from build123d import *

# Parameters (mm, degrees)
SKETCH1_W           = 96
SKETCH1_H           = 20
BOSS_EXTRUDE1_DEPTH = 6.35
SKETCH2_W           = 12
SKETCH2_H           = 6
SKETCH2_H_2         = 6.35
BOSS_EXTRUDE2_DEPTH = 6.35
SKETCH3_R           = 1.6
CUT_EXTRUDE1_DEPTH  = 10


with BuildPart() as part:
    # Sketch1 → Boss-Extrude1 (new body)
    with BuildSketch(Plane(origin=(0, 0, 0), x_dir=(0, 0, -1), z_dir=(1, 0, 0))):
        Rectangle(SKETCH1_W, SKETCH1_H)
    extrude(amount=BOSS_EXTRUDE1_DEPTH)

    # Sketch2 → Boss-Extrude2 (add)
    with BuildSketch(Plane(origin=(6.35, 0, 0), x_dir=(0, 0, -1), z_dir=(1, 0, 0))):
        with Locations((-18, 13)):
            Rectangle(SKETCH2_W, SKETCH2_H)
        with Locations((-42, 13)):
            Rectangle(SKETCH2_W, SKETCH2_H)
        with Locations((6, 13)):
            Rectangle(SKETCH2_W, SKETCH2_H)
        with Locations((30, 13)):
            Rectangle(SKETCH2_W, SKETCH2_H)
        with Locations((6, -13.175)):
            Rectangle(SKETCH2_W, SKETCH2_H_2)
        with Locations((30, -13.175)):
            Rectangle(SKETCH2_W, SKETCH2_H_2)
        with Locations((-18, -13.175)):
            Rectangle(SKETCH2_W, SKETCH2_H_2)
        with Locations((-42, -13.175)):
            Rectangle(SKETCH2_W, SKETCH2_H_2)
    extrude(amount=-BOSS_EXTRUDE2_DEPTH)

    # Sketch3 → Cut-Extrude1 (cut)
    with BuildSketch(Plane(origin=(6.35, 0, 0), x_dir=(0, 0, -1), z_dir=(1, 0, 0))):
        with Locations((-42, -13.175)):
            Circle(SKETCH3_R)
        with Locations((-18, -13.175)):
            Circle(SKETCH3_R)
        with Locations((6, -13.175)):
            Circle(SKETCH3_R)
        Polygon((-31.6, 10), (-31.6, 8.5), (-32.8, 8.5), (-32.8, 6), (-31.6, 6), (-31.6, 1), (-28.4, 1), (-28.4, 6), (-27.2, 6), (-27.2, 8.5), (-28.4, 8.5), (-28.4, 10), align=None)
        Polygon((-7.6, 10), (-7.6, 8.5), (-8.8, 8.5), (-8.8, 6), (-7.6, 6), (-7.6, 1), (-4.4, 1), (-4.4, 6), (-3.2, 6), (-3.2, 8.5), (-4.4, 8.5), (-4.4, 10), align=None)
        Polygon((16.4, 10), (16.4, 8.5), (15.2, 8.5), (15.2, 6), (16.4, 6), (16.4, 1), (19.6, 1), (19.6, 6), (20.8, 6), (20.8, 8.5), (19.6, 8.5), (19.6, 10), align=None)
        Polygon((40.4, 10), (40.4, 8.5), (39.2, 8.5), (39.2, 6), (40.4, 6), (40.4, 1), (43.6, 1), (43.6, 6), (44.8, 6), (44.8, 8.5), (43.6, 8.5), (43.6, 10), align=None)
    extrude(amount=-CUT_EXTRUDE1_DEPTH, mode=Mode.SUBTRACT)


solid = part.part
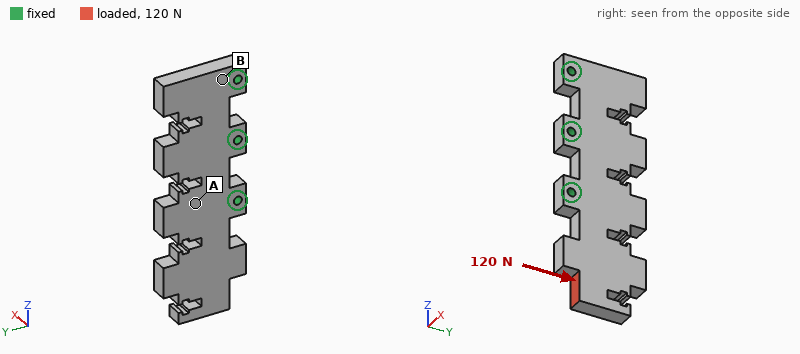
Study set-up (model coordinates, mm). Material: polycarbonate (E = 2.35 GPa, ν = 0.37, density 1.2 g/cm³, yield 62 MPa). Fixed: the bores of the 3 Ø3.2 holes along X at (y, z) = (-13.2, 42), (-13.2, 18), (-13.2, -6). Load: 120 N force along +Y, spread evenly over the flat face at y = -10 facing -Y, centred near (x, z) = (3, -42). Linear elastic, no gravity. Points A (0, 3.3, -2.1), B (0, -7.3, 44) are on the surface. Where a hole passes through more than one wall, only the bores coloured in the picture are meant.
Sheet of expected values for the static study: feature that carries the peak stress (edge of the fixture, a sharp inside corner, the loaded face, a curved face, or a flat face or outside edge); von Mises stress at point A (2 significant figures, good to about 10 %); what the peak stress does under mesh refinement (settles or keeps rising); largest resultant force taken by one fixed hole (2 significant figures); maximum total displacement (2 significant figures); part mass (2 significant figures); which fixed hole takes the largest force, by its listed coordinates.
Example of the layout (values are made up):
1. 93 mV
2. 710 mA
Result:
1. a sharp inside corner
2. 5.2 MPa
3. keeps rising
4. 320 N
5. 1.1 mm
6. 18 g
7. (-13.2, -6)
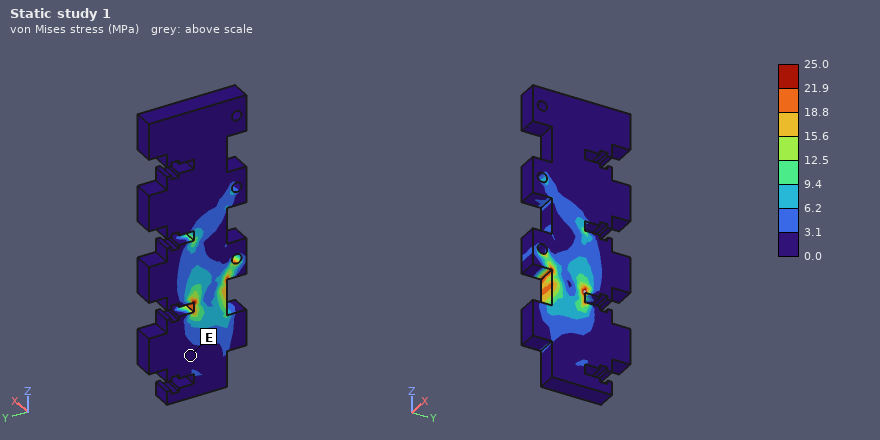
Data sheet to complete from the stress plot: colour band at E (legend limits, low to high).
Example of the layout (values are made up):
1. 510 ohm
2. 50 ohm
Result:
1. 0.0 to 3.1 MPa
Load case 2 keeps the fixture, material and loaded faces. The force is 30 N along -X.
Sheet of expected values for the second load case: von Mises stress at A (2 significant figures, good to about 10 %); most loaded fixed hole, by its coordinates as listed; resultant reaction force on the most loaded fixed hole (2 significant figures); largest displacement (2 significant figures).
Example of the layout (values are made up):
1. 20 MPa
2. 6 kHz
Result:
1. 3.1 MPa
2. (-13.2, -6)
3. 53 N
4. 1.1 mm
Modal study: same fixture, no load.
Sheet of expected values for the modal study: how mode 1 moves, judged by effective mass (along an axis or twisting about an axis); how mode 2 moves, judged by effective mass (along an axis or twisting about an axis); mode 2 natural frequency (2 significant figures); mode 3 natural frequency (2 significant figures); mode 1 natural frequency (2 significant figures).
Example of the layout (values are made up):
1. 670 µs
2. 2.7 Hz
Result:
1. along X
2. along Y
3. 1100 Hz
4. 1200 Hz
5. 560 Hz
